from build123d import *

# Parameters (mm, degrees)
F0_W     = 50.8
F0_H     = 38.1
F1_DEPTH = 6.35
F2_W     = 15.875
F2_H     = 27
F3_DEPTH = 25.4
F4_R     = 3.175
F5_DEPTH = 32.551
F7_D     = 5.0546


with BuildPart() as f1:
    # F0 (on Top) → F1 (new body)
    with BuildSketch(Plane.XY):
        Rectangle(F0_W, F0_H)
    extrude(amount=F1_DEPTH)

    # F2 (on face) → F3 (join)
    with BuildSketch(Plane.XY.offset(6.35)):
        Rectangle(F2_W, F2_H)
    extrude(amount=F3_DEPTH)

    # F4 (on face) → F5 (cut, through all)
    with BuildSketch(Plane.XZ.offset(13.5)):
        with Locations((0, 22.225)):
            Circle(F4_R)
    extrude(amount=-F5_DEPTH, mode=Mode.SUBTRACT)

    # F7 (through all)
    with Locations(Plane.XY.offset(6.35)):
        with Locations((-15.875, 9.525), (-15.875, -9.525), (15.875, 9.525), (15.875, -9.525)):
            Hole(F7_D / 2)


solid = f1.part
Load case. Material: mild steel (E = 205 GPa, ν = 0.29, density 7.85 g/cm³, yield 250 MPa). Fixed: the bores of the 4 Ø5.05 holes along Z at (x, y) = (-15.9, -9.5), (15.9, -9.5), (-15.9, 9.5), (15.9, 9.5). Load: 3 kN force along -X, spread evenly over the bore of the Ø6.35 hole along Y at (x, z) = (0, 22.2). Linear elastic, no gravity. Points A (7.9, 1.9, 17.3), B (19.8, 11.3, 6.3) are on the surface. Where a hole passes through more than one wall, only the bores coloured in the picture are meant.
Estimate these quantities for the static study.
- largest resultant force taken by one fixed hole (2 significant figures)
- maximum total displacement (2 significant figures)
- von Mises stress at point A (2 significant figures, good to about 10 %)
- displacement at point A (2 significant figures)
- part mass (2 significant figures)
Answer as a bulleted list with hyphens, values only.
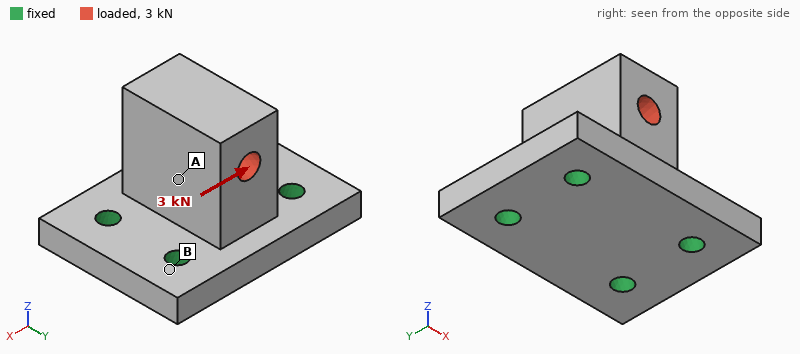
- 1.4 kN
- 15 µm
- 16 MPa
- 7.2 µm
- 170 g
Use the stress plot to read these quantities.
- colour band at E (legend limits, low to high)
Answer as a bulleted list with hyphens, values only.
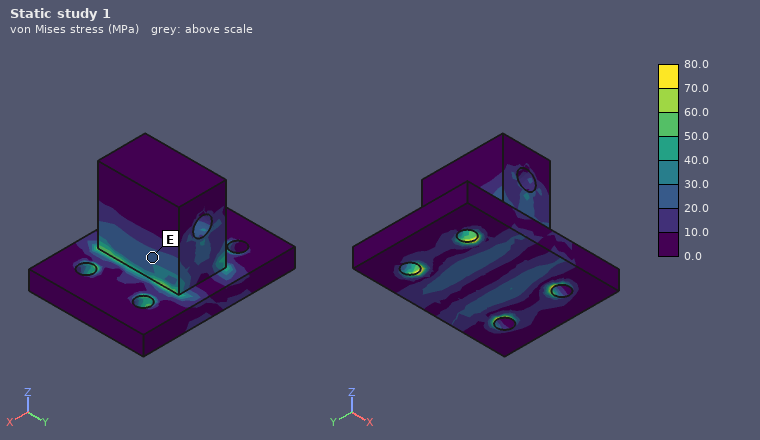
- 20.0 to 30.0 MPa
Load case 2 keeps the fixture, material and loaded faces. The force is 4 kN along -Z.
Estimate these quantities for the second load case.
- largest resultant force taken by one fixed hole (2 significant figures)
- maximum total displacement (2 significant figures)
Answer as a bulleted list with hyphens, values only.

- 1.0 kN
- 3.7 µm
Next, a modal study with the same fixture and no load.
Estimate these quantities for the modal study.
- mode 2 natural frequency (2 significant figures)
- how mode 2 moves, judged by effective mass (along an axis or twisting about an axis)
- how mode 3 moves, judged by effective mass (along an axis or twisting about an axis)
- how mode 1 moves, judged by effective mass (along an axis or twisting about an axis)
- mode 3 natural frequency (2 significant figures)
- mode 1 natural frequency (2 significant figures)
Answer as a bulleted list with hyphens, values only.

- 11 kHz
- along X
- along Z
- along Y
- 18 kHz
- 10 kHz
